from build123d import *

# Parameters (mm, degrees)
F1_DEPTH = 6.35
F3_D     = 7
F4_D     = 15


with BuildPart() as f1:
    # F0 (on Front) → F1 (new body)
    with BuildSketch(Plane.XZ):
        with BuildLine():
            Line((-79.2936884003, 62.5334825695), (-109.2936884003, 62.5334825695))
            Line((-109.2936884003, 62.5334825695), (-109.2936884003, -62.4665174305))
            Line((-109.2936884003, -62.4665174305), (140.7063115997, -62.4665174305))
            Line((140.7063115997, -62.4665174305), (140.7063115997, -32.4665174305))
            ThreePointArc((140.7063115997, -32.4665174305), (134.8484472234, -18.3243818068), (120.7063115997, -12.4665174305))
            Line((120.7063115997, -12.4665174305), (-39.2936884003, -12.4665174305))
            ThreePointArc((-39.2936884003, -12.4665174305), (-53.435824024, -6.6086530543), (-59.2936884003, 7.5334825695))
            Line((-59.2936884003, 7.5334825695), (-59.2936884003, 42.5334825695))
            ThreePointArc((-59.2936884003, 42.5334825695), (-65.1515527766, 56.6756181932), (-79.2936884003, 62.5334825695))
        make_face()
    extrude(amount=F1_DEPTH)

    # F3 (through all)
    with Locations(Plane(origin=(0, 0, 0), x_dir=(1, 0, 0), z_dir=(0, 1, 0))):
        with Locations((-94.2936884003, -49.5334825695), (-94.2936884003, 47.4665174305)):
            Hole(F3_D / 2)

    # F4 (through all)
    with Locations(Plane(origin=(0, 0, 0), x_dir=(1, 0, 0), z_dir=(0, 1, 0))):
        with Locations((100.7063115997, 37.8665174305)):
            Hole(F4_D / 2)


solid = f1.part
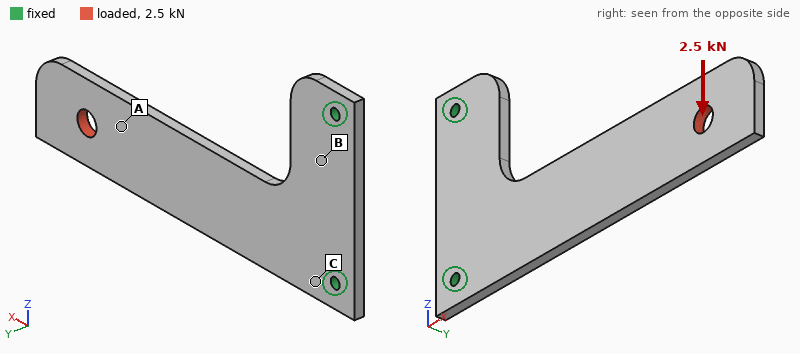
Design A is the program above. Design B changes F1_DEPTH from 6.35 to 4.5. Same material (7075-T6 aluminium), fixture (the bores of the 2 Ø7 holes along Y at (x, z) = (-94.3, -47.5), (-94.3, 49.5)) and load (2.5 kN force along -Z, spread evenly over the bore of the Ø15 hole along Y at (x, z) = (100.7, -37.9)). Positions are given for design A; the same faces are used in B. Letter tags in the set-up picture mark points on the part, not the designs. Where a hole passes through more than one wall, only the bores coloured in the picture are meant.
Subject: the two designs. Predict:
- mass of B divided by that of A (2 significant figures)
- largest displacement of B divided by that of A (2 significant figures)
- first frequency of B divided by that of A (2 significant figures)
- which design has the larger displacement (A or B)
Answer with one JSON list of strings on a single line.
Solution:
["0.71", "1.4", "0.71", "B"]
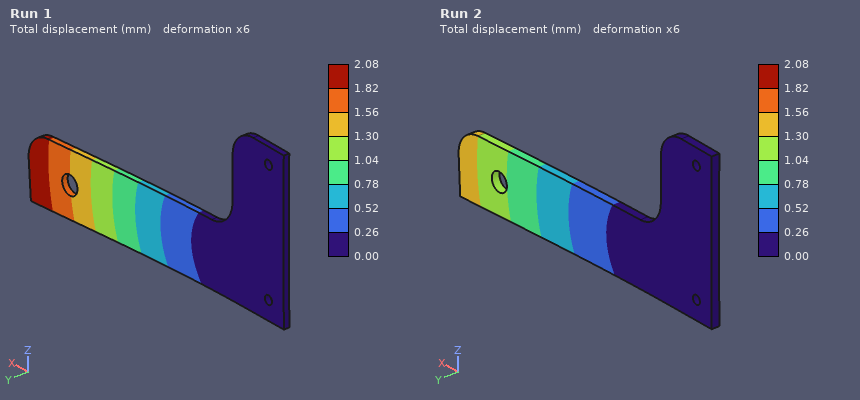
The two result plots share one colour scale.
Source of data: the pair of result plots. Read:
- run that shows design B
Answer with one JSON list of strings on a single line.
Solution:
["Run 1"]
